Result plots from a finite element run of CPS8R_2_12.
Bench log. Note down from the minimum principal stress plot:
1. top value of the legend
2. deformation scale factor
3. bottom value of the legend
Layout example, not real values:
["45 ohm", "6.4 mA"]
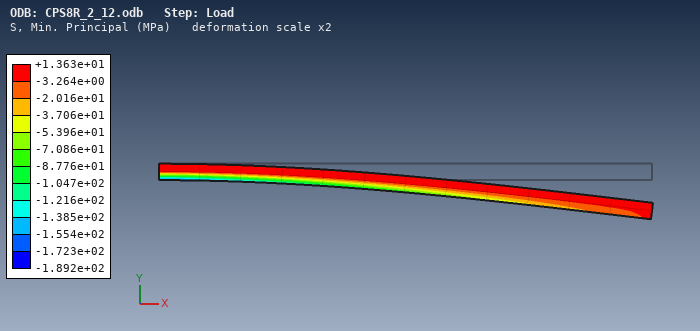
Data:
["+1.363e+01 MPa", "2", "-1.892e+02 MPa"]
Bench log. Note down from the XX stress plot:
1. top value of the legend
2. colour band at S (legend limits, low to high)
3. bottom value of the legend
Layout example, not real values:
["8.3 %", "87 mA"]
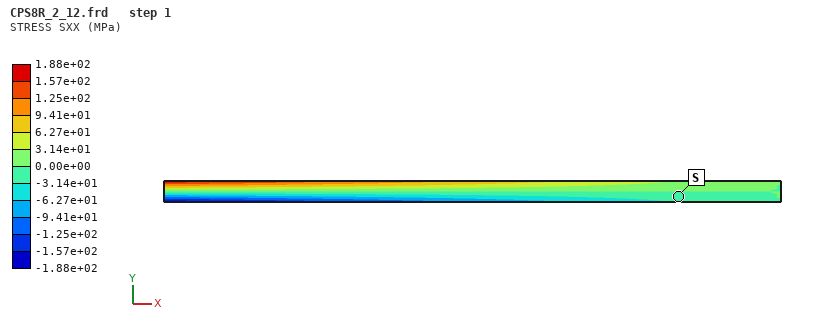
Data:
["1.88e+02 MPa", "-3.14e+01 to 0.00e+00 MPa", "-1.88e+02 MPa"]
